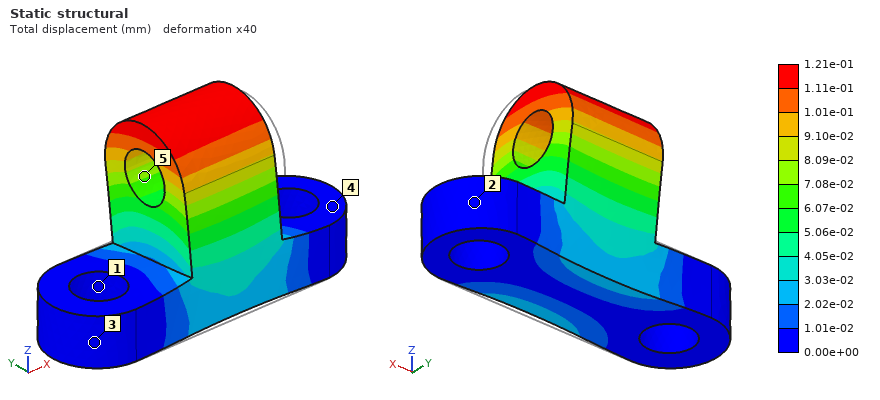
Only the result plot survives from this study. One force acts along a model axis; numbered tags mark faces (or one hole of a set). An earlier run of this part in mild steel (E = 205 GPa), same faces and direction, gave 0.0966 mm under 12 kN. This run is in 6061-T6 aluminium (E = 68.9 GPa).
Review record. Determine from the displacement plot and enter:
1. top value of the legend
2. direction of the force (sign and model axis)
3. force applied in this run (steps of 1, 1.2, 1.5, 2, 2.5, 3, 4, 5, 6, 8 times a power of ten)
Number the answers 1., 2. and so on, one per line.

1. 1.21e-01 mm
2. +Y
3. 5 kN
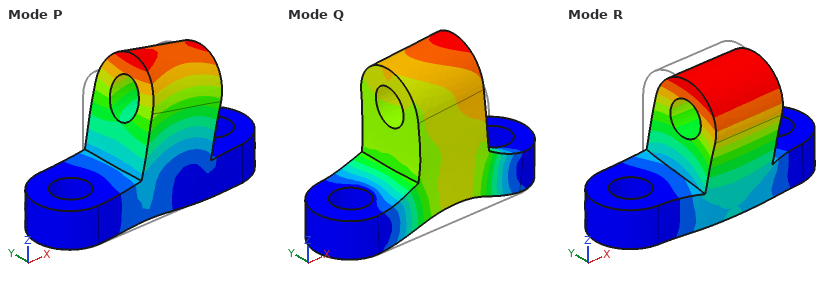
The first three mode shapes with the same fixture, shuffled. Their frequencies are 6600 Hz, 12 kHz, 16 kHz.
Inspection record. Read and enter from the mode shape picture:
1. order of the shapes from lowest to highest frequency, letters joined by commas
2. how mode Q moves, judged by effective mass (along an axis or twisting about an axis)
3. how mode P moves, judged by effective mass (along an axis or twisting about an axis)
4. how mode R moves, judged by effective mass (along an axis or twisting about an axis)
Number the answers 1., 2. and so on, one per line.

1. R, P, Q
2. along Z
3. along X
4. along Y
